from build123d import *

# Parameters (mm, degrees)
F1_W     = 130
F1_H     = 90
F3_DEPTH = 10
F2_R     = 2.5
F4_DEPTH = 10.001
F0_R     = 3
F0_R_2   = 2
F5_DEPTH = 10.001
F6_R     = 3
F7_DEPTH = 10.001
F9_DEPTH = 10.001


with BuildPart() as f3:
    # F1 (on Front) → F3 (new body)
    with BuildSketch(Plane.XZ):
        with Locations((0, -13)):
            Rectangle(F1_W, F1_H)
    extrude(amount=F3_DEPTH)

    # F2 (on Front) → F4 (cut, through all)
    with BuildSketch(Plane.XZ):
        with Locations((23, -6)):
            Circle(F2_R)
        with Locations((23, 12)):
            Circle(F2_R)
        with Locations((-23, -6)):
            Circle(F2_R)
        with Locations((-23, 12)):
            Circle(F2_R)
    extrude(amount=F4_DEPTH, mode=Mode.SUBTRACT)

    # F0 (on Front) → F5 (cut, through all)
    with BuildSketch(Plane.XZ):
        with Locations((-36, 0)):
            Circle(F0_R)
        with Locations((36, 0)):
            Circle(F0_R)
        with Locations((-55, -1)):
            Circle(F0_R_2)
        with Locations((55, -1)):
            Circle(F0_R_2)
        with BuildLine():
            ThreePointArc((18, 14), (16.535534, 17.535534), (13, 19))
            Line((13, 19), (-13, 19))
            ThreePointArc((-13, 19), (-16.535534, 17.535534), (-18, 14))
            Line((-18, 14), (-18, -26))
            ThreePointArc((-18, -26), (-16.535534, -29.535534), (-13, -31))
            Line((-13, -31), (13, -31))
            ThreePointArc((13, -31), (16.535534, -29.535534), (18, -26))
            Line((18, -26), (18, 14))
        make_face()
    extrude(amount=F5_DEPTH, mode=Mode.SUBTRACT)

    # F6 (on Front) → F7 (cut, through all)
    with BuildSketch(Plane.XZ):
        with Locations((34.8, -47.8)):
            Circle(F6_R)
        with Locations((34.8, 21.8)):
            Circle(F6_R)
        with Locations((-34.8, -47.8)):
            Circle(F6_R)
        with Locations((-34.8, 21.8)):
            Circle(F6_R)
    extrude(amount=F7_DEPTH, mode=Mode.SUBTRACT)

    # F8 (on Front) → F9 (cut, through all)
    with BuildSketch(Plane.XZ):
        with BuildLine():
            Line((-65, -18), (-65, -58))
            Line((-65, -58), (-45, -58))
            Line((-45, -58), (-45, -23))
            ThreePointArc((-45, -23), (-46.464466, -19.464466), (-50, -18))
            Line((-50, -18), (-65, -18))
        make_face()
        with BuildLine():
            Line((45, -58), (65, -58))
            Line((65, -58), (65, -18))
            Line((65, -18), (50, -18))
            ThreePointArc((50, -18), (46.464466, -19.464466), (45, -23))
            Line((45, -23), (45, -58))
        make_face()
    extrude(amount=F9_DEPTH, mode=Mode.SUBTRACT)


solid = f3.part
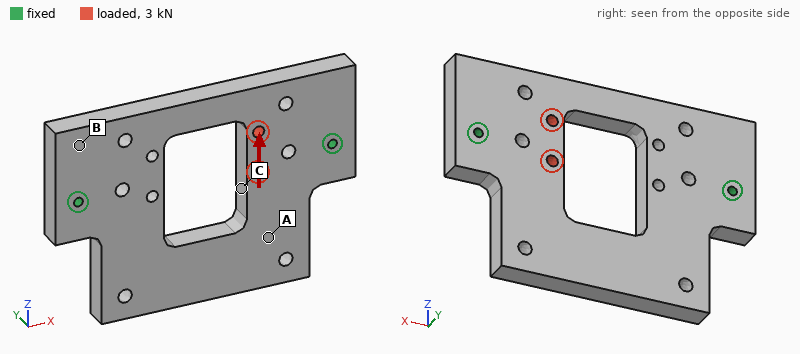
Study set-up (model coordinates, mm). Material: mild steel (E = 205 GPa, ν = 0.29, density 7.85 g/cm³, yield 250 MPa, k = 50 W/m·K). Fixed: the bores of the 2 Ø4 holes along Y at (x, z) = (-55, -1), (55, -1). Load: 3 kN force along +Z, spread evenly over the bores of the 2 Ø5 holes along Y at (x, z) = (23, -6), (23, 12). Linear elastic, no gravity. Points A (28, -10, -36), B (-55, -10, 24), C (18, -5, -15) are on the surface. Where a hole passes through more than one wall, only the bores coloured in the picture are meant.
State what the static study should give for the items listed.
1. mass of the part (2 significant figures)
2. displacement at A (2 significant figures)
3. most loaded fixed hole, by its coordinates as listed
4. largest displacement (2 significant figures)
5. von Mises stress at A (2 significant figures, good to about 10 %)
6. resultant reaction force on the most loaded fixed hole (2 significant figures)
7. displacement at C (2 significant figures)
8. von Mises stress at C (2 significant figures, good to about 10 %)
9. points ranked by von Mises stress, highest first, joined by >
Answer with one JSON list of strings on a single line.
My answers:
["630 g", "4.5 µm", "(55, -1)", "6.7 µm", "7.7 MPa", "2.2 kN", "5.7 µm", "21 MPa", "C > A > B"]
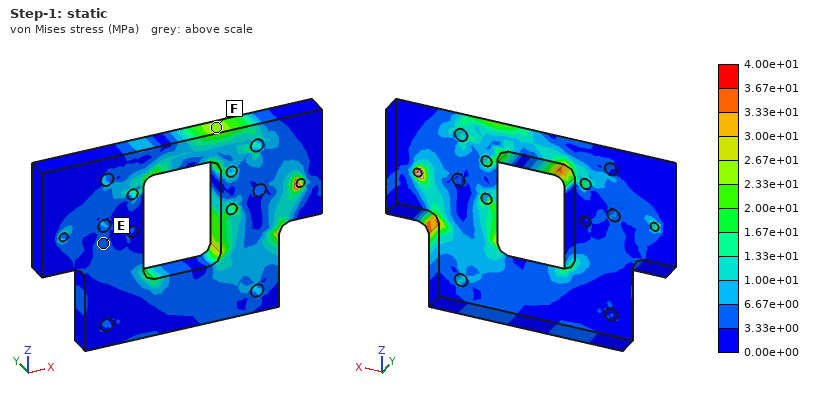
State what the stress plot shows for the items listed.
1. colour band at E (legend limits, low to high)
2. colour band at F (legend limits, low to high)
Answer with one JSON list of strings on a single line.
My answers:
["3.33e+00 to 6.67e+00 MPa", "2.33e+01 to 2.67e+01 MPa"]
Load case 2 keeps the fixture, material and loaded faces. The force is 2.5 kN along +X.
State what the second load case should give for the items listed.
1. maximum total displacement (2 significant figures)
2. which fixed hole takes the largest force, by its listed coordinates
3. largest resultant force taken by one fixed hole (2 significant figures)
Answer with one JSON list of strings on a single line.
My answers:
["2.2 µm", "(55, -1)", "2.1 kN"]
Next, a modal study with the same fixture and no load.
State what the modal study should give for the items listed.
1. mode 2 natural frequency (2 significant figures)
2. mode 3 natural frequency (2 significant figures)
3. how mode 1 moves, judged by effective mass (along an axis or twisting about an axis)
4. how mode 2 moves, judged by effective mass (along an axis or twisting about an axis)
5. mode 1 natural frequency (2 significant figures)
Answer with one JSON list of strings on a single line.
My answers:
["3200 Hz", "3700 Hz", "along Y", "along Y", "1500 Hz"]
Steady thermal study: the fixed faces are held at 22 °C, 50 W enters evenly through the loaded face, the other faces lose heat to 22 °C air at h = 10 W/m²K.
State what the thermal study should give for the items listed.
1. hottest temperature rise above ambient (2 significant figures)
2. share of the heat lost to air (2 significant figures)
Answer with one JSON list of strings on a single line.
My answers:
["81 K", "12 %"]
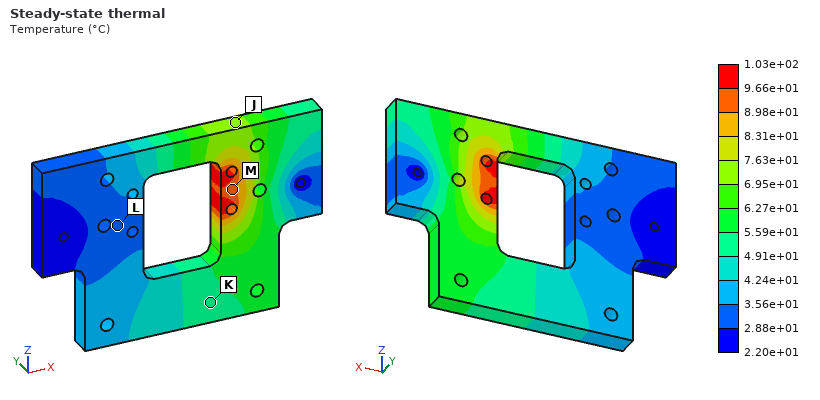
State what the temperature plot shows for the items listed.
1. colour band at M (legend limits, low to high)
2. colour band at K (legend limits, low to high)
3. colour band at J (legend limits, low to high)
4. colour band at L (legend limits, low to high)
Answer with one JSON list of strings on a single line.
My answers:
["8.98e+01 to 9.66e+01 °C", "4.91e+01 to 5.59e+01 °C", "6.95e+01 to 7.63e+01 °C", "2.88e+01 to 3.56e+01 °C"]
